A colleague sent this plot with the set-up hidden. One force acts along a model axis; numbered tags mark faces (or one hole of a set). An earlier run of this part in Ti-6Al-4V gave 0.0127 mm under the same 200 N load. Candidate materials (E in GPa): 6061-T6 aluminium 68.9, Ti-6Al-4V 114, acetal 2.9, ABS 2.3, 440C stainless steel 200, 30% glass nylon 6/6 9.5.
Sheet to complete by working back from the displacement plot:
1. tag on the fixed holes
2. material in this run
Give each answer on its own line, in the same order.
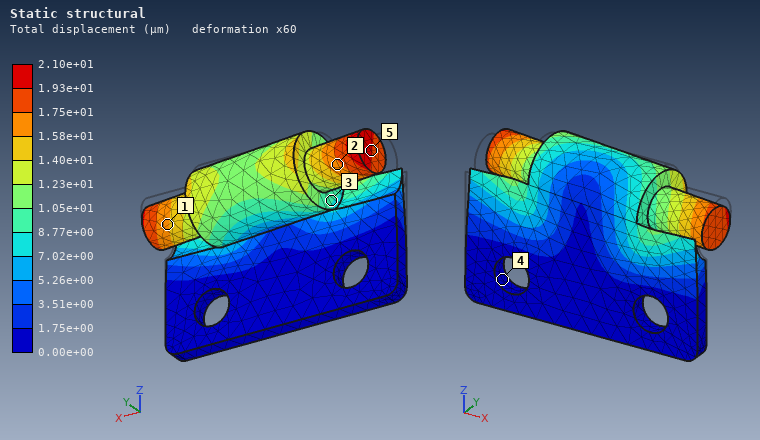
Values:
4
6061-T6 aluminium
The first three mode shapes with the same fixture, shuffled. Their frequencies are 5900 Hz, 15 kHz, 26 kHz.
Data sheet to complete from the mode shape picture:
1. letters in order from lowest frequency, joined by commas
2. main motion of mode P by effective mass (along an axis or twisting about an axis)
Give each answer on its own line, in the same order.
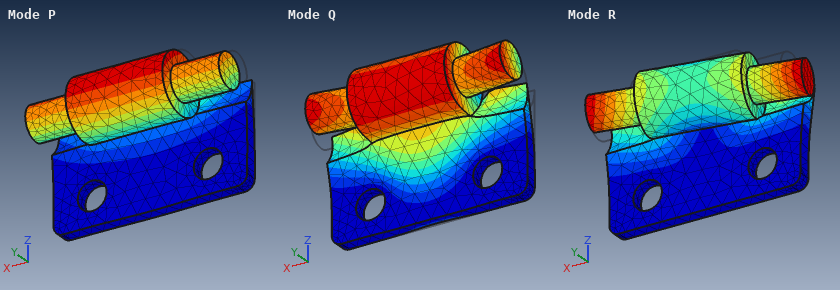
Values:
P, R, Q
along Y
